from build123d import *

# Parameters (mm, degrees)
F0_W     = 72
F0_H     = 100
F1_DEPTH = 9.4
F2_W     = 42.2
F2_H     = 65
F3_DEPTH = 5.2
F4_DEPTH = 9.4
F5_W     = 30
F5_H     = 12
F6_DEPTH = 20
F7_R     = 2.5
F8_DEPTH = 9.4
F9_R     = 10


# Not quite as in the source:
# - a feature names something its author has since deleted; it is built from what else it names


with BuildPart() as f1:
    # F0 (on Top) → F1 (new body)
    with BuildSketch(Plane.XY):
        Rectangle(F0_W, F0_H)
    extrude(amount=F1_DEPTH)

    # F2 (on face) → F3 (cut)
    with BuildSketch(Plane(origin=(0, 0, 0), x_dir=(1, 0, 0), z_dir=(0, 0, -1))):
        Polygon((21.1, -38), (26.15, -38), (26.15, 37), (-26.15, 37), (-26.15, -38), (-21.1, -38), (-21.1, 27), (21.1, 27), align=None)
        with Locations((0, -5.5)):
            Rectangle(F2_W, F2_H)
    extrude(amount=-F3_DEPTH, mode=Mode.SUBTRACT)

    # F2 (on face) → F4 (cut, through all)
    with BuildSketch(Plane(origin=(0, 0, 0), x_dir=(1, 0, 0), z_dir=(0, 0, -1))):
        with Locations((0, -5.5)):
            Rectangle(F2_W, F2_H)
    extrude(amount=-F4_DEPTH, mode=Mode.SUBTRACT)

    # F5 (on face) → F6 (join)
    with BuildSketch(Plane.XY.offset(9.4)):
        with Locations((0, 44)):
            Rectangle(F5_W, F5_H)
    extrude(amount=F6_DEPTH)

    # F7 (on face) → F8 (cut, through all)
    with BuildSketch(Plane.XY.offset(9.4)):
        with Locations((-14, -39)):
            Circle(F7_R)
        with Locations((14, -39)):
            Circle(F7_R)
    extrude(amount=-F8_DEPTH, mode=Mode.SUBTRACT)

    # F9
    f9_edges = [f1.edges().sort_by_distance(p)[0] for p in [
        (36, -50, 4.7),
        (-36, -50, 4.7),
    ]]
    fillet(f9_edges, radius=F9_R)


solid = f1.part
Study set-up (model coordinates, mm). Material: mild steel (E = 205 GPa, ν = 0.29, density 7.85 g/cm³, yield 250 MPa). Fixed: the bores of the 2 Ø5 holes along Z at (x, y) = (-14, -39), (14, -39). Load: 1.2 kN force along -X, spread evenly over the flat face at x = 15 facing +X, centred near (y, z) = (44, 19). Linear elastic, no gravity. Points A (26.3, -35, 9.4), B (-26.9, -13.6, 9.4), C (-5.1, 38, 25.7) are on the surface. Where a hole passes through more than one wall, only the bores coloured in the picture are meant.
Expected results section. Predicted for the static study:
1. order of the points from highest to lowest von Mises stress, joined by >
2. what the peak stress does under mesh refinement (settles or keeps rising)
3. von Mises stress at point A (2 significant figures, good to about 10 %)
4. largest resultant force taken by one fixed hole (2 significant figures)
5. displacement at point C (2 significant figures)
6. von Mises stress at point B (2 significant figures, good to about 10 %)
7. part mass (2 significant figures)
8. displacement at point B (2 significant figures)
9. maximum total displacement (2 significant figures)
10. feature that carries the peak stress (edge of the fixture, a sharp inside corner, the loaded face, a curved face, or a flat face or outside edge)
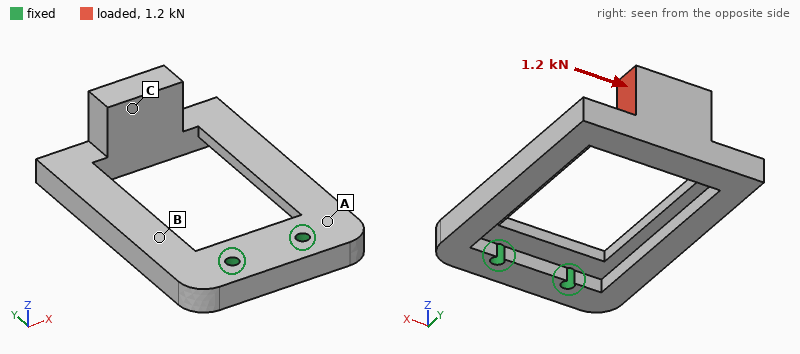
B > A > C
keeps rising
27 MPa
2.7 kN
0.17 mm
42 MPa
330 g
0.033 mm
0.18 mm
a sharp inside corner
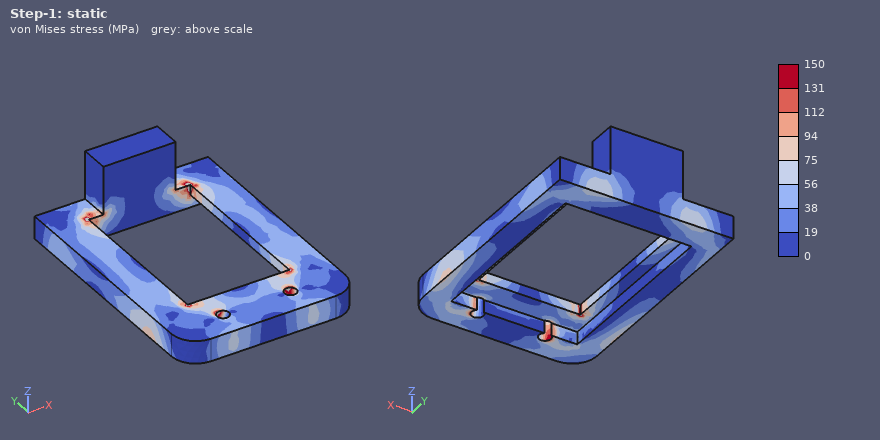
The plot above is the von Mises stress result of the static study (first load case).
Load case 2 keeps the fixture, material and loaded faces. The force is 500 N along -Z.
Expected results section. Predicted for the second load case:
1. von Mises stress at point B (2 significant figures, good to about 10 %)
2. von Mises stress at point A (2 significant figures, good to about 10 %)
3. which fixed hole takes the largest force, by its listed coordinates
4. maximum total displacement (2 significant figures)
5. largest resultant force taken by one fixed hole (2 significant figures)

70 MPa
99 MPa
(14, -39)
0.48 mm
650 N
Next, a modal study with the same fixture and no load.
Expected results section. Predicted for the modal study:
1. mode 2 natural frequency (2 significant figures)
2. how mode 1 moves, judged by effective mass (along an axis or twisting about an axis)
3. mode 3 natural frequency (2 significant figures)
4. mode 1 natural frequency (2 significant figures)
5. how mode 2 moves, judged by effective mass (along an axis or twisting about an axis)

1200 Hz
along Z
1300 Hz
460 Hz
along X
